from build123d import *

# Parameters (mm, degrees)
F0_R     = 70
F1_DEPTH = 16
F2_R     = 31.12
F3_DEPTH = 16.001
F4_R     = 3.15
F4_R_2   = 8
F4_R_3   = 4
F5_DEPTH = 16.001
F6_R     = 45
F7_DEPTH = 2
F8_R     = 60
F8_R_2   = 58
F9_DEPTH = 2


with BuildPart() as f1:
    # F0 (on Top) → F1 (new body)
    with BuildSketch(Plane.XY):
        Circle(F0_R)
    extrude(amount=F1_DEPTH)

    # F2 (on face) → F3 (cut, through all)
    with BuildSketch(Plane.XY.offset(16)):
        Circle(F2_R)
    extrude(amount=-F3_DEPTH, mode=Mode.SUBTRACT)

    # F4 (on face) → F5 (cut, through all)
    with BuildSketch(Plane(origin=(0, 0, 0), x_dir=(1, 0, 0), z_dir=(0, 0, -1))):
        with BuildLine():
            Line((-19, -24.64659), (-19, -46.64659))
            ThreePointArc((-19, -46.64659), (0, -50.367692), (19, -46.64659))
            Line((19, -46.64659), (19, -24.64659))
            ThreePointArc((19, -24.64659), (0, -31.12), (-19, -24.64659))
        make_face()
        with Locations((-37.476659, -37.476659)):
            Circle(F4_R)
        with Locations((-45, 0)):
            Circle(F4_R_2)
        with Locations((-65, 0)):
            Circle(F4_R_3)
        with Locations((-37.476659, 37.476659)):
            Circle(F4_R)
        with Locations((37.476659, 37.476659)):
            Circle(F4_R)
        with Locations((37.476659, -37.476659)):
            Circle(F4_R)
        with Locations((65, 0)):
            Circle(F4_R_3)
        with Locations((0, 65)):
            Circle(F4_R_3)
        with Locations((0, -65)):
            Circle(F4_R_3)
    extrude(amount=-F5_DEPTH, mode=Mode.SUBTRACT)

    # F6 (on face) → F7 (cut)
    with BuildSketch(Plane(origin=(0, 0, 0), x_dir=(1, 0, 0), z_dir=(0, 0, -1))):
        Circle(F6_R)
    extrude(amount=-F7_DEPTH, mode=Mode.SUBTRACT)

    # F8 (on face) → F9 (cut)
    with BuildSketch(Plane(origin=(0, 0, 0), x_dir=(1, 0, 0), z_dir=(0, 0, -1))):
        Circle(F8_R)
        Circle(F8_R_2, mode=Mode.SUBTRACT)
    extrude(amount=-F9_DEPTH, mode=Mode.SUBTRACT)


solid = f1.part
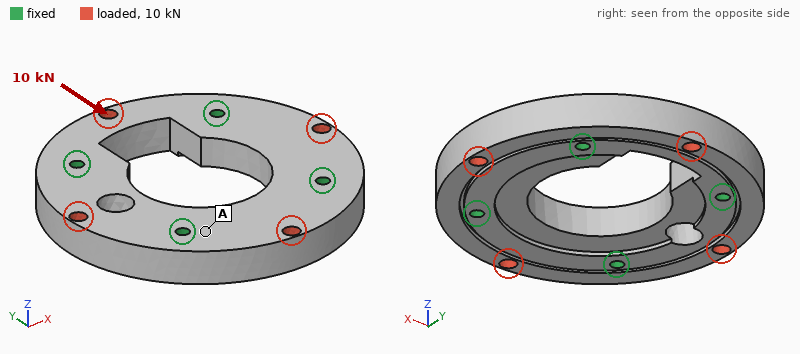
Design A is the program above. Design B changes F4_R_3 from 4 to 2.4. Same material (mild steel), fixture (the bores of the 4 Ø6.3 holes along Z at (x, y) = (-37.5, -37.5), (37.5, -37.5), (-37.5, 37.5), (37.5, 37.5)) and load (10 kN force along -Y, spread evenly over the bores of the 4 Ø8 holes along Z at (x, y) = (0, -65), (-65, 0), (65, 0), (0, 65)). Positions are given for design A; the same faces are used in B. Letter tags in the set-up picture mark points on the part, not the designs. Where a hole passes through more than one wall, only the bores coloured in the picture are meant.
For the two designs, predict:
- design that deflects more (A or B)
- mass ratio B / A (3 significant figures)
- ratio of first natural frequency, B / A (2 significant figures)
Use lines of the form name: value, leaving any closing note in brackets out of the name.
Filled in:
design that deflects more: A
mass ratio B / A: 1.01
ratio of first natural frequency, B / A: 0.99
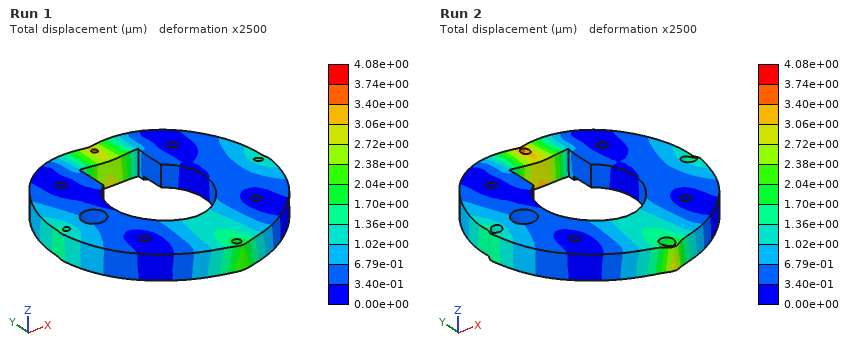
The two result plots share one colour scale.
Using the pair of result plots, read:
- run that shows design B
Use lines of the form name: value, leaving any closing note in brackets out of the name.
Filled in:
run that shows design B: Run 1
